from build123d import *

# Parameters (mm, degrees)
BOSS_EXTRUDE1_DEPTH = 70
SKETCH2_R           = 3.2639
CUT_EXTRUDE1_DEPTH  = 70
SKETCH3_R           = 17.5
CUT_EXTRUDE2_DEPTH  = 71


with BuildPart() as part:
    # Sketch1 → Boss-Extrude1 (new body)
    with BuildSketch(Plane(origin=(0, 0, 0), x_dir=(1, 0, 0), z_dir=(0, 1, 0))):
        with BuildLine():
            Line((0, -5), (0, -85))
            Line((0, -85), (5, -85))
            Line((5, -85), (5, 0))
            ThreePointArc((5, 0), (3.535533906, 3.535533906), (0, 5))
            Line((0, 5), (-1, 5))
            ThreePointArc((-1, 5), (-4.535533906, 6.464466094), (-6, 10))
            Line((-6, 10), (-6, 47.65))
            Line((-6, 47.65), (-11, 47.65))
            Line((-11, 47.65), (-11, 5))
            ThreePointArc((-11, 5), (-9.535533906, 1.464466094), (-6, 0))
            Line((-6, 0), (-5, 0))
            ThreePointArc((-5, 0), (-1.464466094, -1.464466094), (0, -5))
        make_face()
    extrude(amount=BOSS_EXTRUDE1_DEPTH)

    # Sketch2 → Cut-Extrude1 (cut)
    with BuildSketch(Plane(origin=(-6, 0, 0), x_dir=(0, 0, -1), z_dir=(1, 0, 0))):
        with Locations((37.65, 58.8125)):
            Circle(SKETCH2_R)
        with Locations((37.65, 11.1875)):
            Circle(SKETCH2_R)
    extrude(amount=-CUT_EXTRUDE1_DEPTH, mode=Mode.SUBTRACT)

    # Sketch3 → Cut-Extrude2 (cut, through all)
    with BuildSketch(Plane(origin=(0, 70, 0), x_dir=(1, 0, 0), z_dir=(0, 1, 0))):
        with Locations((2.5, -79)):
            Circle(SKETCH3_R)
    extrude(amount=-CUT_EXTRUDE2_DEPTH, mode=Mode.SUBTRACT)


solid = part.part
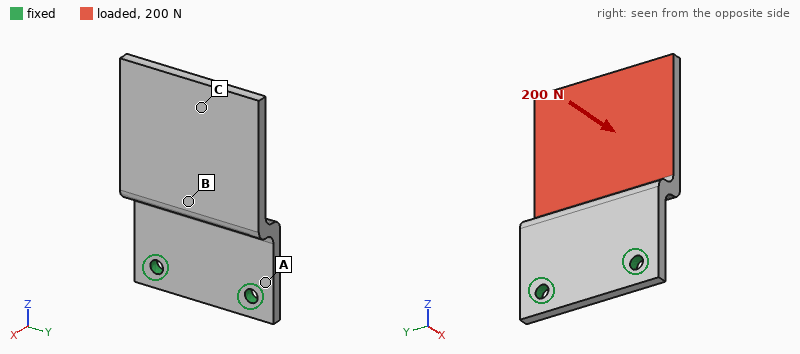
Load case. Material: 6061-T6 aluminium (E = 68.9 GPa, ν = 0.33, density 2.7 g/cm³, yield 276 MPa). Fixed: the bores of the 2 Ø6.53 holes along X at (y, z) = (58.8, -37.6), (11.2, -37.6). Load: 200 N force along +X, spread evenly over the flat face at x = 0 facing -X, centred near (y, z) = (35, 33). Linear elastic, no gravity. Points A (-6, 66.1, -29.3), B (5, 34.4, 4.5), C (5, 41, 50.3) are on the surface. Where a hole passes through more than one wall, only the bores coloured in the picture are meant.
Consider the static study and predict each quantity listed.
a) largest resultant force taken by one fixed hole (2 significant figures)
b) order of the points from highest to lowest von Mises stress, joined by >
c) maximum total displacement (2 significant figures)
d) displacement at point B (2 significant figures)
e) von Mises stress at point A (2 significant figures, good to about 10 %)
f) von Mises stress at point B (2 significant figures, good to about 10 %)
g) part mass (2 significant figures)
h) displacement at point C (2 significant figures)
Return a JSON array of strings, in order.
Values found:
["110 N", "A > B > C", "0.75 mm", "0.22 mm", "45 MPa", "18 MPa", "110 g", "0.64 mm"]
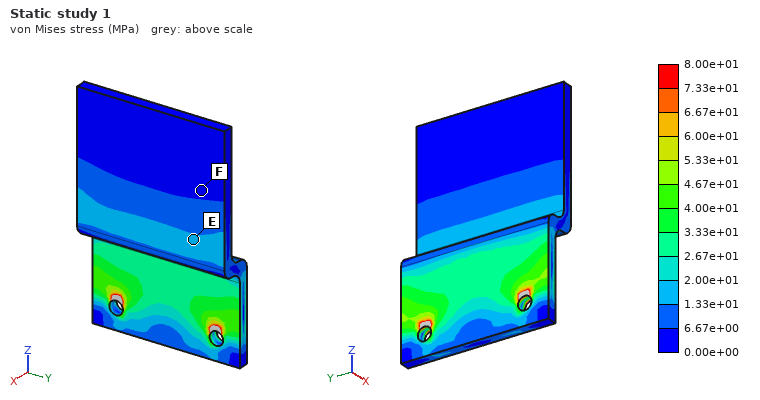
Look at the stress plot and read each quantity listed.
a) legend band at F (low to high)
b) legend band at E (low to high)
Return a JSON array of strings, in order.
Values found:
["0.00e+00 to 6.67e+00 MPa", "1.33e+01 to 2.00e+01 MPa"]
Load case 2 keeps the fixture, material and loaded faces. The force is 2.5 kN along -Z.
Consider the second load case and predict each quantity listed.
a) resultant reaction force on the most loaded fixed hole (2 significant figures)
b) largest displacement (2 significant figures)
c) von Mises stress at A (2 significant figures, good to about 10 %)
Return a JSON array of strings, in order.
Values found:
["1.3 kN", "1.0 mm", "82 MPa"]
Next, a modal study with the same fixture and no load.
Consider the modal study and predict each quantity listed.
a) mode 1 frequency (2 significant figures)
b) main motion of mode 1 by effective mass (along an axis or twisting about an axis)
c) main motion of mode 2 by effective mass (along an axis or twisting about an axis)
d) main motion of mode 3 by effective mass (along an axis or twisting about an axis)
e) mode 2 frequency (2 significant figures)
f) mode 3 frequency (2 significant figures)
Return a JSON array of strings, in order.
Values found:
["410 Hz", "along X", "twisting about Z", "along X", "1400 Hz", "2400 Hz"]
